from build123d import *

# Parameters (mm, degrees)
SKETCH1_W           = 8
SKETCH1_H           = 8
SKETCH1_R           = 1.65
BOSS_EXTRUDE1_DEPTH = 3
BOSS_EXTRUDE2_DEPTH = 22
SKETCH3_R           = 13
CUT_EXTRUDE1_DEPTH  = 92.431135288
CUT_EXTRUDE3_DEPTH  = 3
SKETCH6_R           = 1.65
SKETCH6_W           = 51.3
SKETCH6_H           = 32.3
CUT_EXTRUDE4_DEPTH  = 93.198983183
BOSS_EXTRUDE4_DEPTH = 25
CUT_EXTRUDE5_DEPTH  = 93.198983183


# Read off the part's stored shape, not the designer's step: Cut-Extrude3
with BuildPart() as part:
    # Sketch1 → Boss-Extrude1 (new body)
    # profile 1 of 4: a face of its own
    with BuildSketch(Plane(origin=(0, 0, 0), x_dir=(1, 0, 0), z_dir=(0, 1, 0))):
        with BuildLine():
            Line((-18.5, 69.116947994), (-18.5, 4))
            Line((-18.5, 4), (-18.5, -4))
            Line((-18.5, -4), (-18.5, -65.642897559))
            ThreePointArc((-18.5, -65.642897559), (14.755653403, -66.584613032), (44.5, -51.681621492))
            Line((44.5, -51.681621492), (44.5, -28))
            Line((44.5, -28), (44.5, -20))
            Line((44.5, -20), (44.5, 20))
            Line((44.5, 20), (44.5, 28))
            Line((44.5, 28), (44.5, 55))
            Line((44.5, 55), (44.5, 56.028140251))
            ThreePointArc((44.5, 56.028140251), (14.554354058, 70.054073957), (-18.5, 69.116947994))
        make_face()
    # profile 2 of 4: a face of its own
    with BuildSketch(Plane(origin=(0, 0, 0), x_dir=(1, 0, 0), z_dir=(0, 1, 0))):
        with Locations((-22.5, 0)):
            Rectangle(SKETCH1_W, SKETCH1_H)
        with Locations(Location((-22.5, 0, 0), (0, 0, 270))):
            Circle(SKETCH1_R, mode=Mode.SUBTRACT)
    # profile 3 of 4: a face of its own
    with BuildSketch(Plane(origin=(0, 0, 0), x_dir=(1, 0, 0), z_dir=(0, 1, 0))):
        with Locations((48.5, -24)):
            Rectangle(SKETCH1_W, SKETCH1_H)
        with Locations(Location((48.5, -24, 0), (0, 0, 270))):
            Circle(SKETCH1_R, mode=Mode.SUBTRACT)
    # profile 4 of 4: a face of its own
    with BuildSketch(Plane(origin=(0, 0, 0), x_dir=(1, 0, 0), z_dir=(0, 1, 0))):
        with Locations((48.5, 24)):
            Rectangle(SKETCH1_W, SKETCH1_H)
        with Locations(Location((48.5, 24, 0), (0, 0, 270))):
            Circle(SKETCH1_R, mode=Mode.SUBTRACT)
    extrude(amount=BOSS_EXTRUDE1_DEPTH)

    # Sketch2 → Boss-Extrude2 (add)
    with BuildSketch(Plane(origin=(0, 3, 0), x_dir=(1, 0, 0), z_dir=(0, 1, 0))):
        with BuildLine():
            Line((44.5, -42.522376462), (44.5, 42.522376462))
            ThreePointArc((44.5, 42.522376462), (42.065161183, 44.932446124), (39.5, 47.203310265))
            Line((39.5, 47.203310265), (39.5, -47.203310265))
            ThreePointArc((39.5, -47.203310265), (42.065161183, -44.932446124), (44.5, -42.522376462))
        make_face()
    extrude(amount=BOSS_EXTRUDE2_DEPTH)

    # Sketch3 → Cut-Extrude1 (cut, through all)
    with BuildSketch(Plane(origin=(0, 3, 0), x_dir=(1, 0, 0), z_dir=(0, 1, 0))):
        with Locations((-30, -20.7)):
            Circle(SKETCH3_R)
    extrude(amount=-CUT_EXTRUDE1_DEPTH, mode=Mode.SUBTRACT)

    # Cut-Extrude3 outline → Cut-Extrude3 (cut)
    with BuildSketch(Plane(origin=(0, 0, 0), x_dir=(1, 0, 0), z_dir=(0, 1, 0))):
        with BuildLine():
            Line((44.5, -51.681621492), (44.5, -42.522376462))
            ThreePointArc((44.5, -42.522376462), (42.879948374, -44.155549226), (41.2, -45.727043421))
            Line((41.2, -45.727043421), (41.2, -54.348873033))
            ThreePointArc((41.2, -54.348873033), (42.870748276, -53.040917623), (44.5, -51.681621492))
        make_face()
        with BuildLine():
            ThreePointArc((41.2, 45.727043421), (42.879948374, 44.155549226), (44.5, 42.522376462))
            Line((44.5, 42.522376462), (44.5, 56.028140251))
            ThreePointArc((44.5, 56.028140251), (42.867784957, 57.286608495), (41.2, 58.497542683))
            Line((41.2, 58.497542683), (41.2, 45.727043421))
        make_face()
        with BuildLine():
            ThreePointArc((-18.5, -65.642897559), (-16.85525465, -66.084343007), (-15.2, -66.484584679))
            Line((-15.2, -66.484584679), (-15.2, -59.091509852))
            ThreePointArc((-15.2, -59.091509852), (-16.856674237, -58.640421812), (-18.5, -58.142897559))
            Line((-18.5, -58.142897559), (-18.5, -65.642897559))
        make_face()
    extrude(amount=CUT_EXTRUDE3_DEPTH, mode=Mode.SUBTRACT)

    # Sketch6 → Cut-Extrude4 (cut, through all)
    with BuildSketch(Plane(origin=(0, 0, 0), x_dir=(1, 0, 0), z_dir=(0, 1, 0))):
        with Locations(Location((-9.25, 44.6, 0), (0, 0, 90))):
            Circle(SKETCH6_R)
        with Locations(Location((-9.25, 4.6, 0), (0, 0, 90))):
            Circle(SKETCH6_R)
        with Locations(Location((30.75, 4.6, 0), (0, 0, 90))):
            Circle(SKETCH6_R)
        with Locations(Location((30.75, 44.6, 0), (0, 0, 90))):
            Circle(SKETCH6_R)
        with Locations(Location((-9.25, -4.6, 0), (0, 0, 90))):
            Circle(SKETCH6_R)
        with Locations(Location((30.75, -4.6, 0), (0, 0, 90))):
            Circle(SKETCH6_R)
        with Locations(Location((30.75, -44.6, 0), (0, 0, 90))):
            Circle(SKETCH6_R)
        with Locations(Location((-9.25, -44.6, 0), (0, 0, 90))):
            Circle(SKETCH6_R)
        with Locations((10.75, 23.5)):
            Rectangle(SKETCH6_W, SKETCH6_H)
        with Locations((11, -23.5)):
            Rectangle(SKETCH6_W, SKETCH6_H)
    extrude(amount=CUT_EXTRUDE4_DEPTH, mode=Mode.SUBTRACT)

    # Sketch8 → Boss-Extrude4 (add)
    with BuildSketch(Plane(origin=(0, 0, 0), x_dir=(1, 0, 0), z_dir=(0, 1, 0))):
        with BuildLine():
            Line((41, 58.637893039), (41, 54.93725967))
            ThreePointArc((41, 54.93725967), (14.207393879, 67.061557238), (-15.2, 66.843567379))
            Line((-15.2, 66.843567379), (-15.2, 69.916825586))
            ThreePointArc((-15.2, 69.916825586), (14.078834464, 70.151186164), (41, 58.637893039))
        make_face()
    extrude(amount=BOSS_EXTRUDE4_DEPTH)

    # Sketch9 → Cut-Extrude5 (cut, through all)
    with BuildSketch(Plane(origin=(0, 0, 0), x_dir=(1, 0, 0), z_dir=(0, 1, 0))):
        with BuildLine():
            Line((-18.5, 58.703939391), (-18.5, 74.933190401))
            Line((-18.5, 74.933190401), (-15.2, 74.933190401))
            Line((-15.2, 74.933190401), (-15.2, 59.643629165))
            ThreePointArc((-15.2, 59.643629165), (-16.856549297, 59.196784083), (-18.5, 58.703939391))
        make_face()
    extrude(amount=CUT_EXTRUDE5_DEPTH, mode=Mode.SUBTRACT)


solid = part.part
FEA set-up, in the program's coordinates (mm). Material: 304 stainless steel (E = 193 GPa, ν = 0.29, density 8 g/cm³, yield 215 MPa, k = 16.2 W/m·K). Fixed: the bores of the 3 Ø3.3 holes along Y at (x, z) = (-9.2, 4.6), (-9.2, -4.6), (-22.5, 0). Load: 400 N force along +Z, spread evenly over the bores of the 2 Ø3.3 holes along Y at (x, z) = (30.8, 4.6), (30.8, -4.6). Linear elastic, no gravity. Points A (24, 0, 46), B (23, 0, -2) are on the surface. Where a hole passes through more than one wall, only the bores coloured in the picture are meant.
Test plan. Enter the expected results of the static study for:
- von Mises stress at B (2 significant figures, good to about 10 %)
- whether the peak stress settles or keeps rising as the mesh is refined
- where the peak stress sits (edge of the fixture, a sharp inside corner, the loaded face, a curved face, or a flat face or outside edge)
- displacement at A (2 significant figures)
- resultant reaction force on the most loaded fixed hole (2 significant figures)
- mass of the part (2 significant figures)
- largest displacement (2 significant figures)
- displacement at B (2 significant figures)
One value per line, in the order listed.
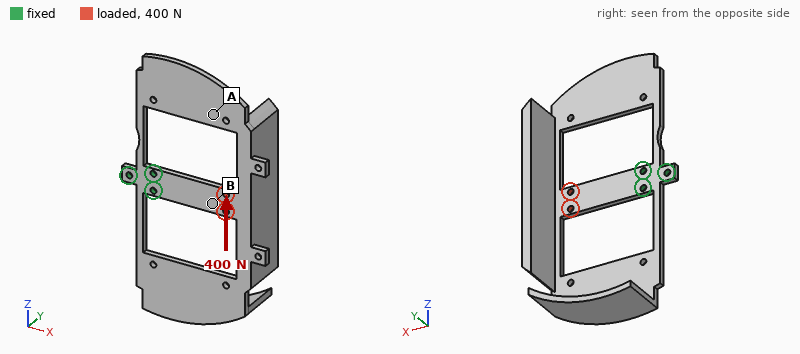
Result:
22 MPa
keeps rising
edge of the fixture
0.076 mm
1.5 kN
230 g
0.10 mm
0.038 mm
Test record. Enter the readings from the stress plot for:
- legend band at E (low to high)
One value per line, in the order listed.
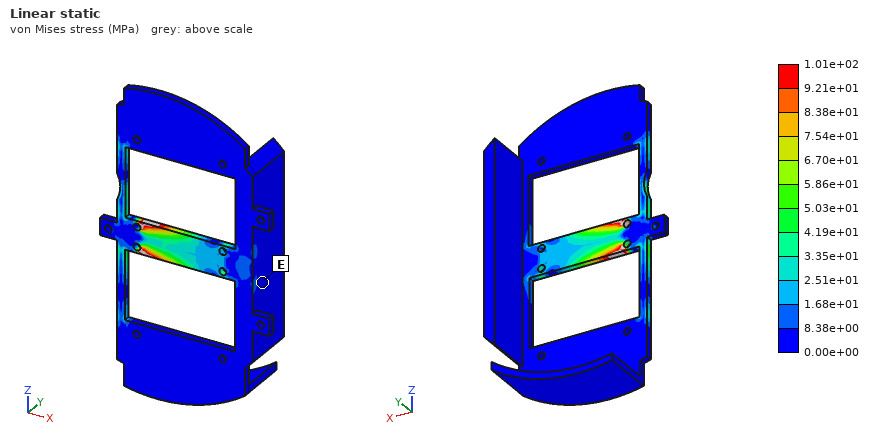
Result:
0.00e+00 to 8.38e+00 MPa
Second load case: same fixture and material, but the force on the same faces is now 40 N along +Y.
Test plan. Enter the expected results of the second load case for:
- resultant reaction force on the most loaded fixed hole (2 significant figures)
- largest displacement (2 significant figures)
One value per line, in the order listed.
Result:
30 N
0.17 mm
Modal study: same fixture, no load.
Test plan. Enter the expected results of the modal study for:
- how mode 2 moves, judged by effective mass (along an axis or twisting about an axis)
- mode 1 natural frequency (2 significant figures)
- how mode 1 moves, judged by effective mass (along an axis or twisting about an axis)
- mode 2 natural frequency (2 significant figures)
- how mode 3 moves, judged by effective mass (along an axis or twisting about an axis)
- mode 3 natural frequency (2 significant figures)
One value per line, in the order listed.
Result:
along Y
150 Hz
along Y
200 Hz
along Y
440 Hz
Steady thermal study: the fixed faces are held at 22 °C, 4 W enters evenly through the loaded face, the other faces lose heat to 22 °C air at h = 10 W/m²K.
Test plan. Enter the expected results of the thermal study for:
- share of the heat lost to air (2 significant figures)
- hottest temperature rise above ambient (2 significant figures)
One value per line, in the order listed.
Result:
72 %
70 K
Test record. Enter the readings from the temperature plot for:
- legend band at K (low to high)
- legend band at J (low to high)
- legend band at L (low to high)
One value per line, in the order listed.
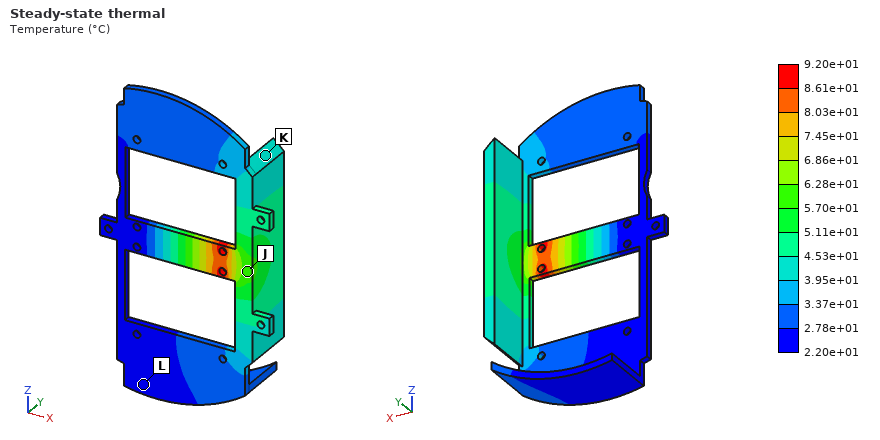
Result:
3.95e+01 to 4.53e+01 °C
5.70e+01 to 6.28e+01 °C
2.20e+01 to 2.78e+01 °C
